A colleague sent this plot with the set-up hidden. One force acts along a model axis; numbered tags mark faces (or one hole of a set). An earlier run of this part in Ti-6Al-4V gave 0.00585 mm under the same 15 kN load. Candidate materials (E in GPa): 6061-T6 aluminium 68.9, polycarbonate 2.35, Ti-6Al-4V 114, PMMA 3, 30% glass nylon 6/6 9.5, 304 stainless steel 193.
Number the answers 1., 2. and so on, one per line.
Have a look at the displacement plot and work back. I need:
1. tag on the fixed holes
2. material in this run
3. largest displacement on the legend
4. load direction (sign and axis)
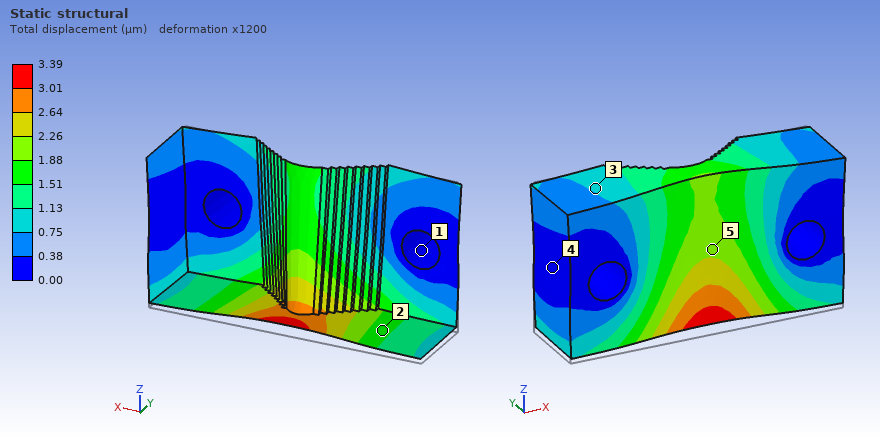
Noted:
1. 1
2. 304 stainless steel
3. 3.39 µm
4. +Z
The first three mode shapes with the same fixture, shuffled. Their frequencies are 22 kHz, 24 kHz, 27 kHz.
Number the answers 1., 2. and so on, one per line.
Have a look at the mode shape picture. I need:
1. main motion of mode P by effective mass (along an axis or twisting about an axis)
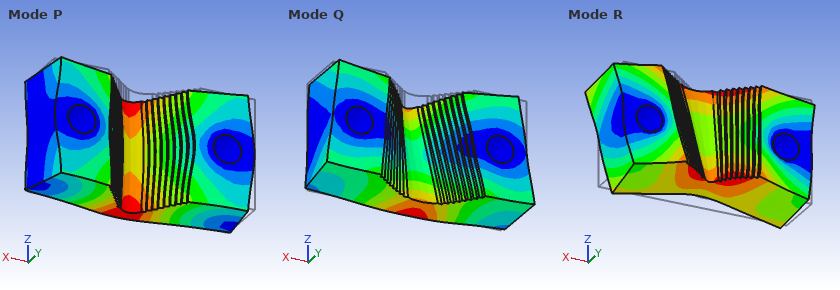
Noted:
1. along Y
